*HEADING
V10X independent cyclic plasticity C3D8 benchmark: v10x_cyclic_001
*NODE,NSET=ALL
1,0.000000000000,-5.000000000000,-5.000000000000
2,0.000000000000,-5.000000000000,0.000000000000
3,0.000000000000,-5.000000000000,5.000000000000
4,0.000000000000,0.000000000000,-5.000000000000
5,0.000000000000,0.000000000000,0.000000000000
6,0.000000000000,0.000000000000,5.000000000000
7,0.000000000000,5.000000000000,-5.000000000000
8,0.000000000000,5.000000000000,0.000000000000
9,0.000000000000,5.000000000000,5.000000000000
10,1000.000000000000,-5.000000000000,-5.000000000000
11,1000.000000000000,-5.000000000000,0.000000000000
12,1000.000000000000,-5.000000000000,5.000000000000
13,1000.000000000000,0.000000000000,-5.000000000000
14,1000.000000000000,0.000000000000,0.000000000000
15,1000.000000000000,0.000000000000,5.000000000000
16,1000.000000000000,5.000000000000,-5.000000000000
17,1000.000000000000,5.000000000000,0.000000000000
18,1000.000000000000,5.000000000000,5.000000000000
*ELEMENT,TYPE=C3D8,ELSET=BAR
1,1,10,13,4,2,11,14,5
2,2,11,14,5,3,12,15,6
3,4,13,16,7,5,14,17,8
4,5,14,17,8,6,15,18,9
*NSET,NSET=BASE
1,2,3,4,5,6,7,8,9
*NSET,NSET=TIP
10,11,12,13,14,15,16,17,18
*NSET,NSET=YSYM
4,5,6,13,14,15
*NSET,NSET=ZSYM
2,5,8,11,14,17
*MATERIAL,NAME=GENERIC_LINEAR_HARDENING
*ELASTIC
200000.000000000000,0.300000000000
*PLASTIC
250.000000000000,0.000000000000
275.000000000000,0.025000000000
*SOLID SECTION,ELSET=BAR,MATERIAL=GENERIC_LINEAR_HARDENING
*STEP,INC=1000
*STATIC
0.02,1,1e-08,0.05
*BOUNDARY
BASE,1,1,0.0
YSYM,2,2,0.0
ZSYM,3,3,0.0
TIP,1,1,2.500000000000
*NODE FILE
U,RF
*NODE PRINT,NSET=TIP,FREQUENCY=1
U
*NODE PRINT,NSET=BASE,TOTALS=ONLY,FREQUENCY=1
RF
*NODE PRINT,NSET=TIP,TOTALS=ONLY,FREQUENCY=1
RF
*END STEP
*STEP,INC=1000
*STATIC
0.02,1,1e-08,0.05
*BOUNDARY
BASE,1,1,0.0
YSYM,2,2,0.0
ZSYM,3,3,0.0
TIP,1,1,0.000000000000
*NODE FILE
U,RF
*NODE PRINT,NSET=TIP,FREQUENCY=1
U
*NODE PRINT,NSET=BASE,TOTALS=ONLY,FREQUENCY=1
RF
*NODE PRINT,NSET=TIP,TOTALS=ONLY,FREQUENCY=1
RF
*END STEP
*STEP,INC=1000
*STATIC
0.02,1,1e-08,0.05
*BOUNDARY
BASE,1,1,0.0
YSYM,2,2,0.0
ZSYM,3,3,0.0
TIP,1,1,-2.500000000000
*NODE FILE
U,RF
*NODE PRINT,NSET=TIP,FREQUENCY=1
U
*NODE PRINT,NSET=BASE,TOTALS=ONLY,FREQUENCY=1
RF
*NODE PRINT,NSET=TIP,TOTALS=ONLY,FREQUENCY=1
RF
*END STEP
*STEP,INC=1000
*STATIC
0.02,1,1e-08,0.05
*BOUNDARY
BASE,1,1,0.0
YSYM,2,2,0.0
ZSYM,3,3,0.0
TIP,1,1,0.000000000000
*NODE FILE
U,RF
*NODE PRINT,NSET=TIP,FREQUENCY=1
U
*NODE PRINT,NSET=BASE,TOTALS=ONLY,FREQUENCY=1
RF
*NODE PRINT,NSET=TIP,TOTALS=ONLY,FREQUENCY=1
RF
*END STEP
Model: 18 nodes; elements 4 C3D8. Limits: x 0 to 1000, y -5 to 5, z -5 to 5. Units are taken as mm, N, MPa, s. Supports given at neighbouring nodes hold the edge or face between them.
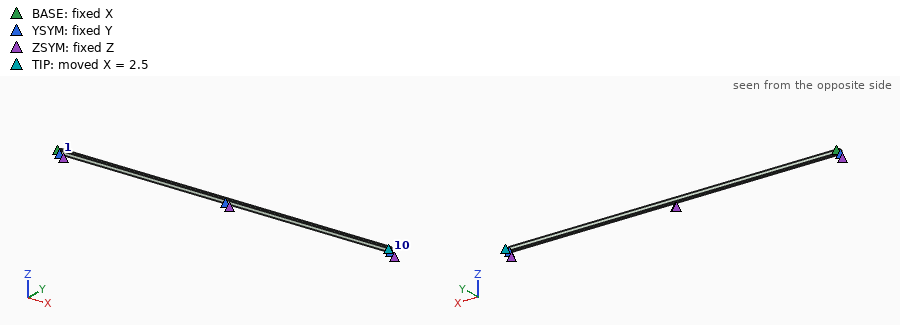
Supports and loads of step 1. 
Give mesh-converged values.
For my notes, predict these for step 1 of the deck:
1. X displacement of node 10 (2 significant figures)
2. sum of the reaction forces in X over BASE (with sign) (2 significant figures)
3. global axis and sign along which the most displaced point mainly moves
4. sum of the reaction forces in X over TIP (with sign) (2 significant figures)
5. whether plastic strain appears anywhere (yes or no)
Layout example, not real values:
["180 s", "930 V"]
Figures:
["2.5 mm", "-25000 N", "+X", "25000 N", "yes"]
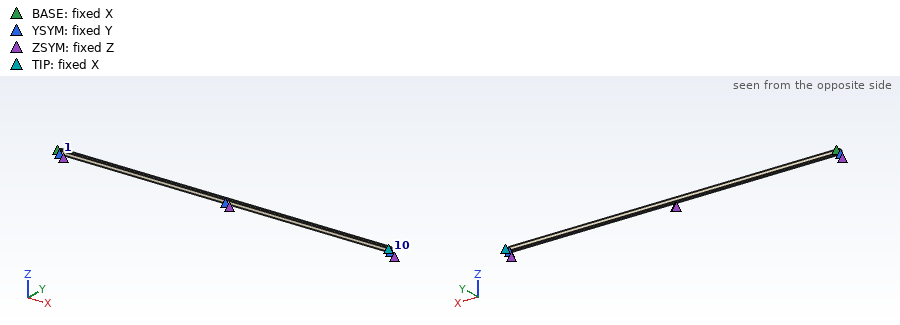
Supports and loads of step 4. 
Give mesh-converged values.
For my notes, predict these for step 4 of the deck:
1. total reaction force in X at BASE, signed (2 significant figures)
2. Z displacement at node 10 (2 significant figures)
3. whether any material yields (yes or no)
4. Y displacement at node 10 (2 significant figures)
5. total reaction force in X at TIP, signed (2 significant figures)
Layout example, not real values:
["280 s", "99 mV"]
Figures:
["-25000 N", "-0.0012 mm", "yes", "-0.0012 mm", "25000 N"]
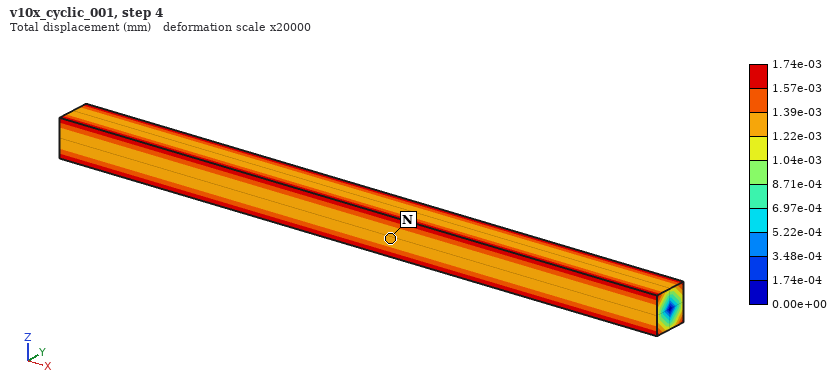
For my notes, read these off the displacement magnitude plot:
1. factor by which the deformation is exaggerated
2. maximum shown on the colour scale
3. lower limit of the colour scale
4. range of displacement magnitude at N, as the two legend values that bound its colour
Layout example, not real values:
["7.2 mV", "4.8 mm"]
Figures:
["20000", "1.74e-03 mm", "0.00e+00 mm", "1.22e-03 to 1.39e-03 mm"]
